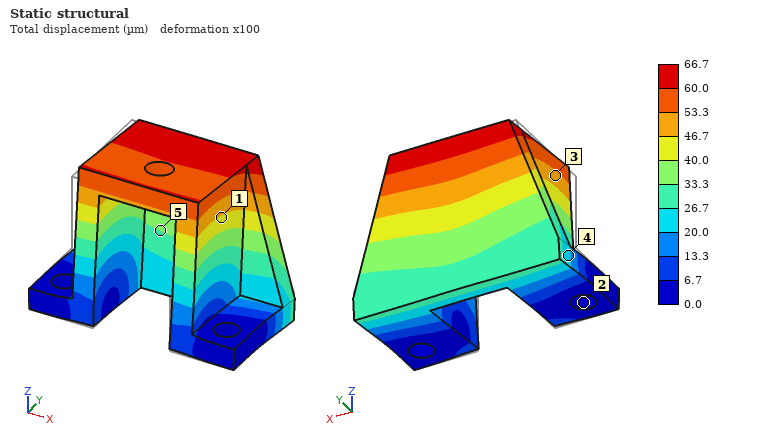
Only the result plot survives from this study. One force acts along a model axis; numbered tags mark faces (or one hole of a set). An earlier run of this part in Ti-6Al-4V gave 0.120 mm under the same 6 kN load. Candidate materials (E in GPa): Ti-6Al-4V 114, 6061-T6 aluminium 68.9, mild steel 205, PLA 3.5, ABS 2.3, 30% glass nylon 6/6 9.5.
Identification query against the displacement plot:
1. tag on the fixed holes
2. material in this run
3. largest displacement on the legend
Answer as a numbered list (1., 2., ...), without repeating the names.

1. 2
2. mild steel
3. 66.7 µm
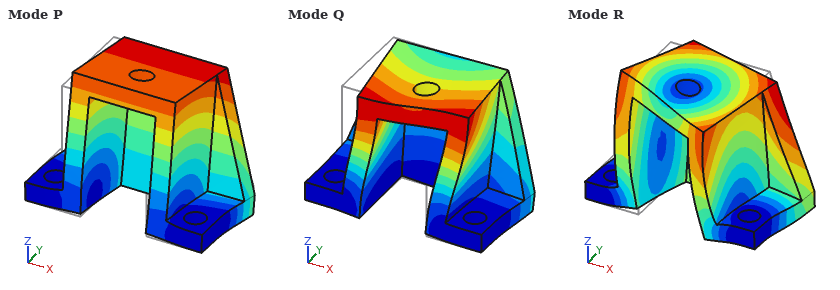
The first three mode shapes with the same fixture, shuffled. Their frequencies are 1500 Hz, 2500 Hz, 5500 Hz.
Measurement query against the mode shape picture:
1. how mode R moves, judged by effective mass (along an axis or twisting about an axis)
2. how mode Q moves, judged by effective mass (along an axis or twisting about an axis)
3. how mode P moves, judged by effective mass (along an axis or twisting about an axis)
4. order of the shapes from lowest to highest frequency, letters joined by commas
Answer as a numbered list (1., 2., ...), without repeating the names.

1. along X
2. along X
3. along Y
4. P, Q, R
